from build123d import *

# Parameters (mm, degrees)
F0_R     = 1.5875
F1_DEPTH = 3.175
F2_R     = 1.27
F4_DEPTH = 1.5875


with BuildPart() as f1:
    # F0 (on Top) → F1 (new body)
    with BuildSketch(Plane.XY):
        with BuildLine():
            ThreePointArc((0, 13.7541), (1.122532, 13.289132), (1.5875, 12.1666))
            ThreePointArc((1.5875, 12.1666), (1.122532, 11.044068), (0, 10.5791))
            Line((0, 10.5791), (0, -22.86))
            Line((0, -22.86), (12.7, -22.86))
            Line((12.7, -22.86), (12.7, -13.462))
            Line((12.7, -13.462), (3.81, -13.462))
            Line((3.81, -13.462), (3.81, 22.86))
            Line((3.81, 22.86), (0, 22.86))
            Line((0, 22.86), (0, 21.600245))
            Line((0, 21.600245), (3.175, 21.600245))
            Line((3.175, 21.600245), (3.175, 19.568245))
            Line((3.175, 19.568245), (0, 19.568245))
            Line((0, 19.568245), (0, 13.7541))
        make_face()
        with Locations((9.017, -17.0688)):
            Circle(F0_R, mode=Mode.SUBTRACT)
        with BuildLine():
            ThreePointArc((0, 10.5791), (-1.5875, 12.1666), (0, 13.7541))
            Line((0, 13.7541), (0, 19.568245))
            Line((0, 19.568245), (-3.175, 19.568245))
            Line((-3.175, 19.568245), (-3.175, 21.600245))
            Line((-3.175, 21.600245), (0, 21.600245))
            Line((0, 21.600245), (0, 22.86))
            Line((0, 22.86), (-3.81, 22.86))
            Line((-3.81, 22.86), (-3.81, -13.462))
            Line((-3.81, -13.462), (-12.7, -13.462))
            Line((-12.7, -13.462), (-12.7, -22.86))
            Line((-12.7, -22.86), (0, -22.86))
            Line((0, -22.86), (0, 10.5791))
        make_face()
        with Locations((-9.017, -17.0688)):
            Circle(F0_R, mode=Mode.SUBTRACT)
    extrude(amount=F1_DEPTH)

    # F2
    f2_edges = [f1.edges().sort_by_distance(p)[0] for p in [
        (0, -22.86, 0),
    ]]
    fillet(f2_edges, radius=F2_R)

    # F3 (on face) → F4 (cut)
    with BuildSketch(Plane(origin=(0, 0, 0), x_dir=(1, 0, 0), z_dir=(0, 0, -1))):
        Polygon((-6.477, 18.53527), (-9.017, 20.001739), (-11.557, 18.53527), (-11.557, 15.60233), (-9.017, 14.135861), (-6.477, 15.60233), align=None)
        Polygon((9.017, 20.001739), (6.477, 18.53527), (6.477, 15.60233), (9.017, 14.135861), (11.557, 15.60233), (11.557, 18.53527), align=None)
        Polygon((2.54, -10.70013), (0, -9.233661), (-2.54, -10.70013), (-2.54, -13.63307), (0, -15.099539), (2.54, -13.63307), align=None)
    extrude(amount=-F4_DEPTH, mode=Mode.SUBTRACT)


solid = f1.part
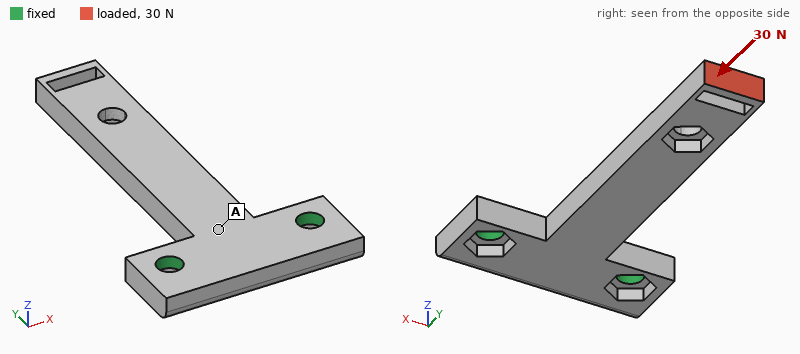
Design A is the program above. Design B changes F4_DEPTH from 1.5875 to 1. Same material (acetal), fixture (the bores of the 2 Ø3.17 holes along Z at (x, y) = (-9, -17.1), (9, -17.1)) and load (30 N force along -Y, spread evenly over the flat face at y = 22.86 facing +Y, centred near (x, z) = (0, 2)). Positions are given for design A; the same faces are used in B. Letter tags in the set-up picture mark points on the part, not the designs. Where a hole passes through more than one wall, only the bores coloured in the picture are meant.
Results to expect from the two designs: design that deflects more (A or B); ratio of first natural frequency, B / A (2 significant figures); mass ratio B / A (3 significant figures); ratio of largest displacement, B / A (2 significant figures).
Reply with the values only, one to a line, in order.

A
1.0
1.02
0.85
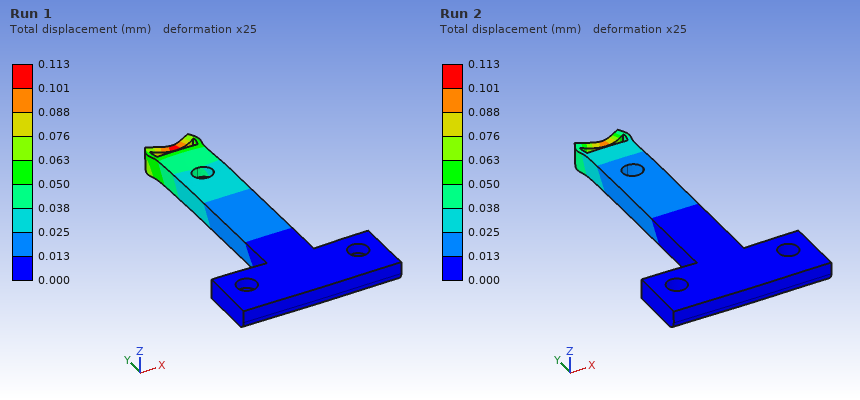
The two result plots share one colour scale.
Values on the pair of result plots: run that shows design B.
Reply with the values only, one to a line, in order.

Run 2
